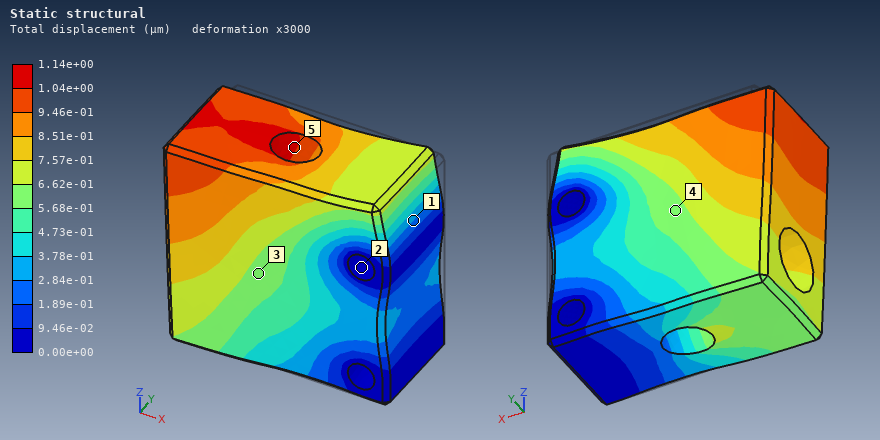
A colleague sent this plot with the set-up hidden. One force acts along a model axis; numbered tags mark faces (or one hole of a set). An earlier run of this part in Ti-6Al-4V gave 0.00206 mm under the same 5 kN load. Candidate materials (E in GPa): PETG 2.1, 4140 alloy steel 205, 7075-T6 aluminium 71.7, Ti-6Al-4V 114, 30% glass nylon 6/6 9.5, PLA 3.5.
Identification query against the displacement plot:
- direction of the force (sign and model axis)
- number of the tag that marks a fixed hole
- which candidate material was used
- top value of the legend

-X
2
4140 alloy steel
1.14e+00 µm
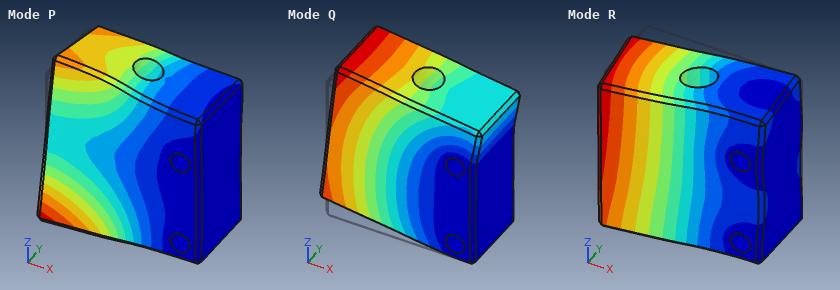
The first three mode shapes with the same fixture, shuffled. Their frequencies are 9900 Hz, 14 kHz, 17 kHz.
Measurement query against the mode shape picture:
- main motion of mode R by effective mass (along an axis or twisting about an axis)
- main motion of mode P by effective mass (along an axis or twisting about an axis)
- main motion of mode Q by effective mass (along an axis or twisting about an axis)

along Y
twisting about X
along Z
